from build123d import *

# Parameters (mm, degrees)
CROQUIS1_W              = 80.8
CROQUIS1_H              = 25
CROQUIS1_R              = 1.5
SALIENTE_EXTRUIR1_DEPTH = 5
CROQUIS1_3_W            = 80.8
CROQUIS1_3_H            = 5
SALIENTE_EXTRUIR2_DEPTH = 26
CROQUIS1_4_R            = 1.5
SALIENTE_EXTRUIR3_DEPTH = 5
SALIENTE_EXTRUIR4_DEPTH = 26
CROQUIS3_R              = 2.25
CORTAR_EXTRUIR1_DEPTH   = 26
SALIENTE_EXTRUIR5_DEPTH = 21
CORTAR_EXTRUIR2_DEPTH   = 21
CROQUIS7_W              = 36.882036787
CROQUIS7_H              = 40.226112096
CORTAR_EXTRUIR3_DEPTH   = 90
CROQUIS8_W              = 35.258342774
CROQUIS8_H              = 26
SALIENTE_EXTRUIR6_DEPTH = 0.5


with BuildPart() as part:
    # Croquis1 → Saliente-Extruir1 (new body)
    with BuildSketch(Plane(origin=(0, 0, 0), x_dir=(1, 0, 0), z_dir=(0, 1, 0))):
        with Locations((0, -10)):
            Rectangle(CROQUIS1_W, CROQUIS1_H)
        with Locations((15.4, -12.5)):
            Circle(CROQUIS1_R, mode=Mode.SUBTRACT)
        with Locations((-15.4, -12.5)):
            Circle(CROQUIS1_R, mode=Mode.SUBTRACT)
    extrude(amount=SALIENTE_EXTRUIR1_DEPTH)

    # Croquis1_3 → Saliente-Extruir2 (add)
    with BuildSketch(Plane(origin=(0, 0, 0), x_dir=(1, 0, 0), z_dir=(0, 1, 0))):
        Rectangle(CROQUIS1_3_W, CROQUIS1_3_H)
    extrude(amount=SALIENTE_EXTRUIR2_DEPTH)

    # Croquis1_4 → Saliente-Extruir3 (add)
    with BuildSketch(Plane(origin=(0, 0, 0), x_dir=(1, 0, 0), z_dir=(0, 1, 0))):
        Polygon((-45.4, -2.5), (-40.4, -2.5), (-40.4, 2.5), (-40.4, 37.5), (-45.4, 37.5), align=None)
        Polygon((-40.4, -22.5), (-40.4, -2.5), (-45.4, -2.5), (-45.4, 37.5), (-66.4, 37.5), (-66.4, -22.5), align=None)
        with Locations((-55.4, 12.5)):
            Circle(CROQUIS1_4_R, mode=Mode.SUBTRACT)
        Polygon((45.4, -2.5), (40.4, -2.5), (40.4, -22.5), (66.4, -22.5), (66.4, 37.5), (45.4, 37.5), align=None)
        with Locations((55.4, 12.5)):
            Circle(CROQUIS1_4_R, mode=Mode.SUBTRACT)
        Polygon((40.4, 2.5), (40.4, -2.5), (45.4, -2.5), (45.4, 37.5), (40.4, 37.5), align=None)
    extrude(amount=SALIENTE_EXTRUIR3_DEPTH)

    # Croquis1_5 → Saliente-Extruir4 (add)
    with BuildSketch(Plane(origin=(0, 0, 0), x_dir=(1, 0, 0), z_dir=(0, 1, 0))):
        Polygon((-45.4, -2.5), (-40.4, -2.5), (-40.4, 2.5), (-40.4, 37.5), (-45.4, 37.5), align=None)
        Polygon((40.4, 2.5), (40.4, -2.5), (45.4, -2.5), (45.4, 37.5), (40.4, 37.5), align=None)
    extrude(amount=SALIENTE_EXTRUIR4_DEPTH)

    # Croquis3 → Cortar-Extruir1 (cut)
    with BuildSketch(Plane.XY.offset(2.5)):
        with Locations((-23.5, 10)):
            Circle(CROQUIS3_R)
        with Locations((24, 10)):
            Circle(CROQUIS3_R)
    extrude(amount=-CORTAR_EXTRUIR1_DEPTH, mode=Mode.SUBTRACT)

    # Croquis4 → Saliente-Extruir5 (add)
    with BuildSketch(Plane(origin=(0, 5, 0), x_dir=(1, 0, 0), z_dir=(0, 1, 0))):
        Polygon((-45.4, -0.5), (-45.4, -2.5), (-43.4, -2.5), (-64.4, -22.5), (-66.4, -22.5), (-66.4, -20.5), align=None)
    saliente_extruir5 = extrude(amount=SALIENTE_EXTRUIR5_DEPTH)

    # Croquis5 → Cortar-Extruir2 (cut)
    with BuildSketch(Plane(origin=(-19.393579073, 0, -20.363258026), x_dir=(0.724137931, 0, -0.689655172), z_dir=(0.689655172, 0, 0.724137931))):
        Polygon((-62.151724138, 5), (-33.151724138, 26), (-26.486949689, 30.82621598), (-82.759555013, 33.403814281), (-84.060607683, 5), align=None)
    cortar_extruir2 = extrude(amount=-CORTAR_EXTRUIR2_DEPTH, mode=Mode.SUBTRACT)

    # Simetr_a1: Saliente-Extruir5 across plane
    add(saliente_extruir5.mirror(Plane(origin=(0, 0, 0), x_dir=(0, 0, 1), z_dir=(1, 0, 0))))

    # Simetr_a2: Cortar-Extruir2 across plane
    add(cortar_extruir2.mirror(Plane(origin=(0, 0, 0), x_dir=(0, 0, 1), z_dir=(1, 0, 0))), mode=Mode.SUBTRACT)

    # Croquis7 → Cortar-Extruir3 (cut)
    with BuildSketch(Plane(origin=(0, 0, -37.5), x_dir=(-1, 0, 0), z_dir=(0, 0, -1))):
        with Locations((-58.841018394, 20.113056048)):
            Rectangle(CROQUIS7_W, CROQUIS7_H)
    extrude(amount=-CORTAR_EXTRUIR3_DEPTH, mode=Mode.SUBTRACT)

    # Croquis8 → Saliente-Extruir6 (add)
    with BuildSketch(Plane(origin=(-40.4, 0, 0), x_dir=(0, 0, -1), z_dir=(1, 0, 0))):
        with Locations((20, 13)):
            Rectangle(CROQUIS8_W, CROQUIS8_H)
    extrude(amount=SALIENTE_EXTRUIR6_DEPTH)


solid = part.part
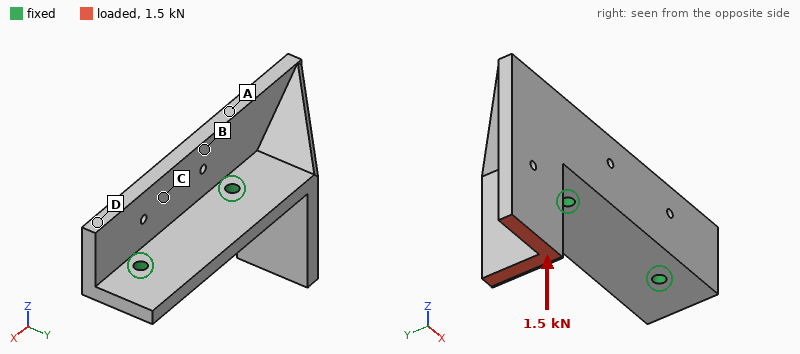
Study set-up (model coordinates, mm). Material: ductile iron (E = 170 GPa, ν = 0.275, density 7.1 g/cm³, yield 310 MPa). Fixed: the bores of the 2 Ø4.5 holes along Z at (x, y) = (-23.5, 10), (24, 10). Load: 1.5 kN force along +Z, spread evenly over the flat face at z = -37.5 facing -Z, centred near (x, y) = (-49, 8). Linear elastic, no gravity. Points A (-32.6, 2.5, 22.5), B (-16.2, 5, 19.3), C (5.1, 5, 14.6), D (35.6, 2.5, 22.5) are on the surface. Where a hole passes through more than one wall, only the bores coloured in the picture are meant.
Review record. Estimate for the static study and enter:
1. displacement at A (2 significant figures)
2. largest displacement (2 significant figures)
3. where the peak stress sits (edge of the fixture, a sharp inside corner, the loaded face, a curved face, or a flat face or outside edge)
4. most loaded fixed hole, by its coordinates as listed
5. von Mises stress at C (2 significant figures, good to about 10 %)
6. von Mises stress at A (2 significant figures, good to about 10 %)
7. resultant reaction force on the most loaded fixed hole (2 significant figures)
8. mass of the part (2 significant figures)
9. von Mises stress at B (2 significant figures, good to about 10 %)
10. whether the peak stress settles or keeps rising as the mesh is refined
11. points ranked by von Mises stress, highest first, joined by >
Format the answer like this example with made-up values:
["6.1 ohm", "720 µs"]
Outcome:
["18 µm", "59 µm", "edge of the fixture", "(-23.5, 10)", "19 MPa", "38 MPa", "2.3 kN", "220 g", "28 MPa", "keeps rising", "A > B > C > D"]
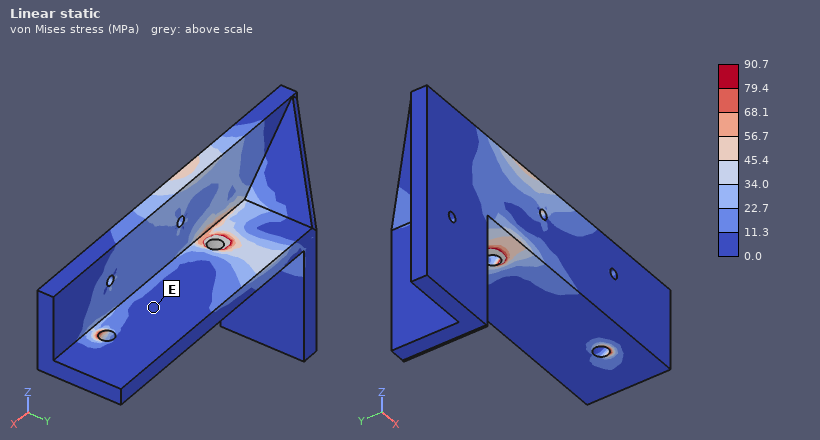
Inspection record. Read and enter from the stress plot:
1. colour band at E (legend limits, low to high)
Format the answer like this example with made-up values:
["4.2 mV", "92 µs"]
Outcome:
["0.0 to 11.3 MPa"]
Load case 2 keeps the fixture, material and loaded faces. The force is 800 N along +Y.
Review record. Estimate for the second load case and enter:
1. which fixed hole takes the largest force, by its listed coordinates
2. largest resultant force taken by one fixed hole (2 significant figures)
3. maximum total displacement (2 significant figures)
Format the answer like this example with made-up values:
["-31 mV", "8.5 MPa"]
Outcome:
["(-23.5, 10)", "1.1 kN", "0.22 mm"]
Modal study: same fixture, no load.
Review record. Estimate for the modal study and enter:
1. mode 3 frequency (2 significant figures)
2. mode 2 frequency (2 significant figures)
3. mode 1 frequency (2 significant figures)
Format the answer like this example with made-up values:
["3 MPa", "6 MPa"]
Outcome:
["4000 Hz", "2700 Hz", "1900 Hz"]
